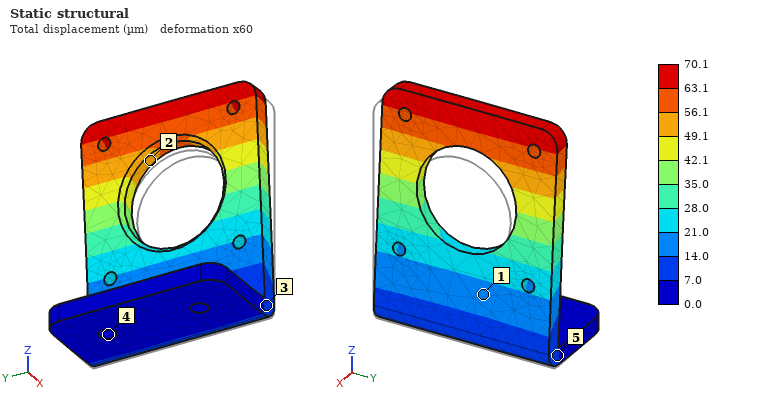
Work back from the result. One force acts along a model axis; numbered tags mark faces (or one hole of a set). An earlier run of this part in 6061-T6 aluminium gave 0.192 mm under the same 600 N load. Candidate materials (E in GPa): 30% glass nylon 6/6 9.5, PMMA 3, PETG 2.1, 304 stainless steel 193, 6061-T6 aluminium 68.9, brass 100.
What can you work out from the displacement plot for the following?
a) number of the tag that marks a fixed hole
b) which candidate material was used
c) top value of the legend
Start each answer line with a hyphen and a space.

- 4
- 304 stainless steel
- 70.1 µm
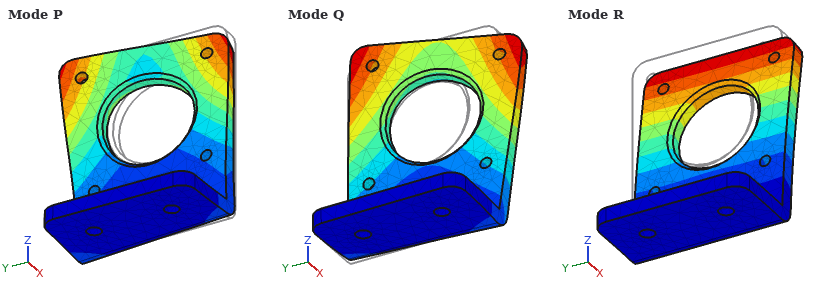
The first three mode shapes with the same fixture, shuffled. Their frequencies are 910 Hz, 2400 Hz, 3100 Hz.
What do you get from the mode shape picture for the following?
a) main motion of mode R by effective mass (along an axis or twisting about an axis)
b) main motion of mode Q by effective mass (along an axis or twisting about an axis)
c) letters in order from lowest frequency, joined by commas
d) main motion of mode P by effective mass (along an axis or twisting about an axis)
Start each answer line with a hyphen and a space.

- along X
- along Y
- R, Q, P
- along Y
